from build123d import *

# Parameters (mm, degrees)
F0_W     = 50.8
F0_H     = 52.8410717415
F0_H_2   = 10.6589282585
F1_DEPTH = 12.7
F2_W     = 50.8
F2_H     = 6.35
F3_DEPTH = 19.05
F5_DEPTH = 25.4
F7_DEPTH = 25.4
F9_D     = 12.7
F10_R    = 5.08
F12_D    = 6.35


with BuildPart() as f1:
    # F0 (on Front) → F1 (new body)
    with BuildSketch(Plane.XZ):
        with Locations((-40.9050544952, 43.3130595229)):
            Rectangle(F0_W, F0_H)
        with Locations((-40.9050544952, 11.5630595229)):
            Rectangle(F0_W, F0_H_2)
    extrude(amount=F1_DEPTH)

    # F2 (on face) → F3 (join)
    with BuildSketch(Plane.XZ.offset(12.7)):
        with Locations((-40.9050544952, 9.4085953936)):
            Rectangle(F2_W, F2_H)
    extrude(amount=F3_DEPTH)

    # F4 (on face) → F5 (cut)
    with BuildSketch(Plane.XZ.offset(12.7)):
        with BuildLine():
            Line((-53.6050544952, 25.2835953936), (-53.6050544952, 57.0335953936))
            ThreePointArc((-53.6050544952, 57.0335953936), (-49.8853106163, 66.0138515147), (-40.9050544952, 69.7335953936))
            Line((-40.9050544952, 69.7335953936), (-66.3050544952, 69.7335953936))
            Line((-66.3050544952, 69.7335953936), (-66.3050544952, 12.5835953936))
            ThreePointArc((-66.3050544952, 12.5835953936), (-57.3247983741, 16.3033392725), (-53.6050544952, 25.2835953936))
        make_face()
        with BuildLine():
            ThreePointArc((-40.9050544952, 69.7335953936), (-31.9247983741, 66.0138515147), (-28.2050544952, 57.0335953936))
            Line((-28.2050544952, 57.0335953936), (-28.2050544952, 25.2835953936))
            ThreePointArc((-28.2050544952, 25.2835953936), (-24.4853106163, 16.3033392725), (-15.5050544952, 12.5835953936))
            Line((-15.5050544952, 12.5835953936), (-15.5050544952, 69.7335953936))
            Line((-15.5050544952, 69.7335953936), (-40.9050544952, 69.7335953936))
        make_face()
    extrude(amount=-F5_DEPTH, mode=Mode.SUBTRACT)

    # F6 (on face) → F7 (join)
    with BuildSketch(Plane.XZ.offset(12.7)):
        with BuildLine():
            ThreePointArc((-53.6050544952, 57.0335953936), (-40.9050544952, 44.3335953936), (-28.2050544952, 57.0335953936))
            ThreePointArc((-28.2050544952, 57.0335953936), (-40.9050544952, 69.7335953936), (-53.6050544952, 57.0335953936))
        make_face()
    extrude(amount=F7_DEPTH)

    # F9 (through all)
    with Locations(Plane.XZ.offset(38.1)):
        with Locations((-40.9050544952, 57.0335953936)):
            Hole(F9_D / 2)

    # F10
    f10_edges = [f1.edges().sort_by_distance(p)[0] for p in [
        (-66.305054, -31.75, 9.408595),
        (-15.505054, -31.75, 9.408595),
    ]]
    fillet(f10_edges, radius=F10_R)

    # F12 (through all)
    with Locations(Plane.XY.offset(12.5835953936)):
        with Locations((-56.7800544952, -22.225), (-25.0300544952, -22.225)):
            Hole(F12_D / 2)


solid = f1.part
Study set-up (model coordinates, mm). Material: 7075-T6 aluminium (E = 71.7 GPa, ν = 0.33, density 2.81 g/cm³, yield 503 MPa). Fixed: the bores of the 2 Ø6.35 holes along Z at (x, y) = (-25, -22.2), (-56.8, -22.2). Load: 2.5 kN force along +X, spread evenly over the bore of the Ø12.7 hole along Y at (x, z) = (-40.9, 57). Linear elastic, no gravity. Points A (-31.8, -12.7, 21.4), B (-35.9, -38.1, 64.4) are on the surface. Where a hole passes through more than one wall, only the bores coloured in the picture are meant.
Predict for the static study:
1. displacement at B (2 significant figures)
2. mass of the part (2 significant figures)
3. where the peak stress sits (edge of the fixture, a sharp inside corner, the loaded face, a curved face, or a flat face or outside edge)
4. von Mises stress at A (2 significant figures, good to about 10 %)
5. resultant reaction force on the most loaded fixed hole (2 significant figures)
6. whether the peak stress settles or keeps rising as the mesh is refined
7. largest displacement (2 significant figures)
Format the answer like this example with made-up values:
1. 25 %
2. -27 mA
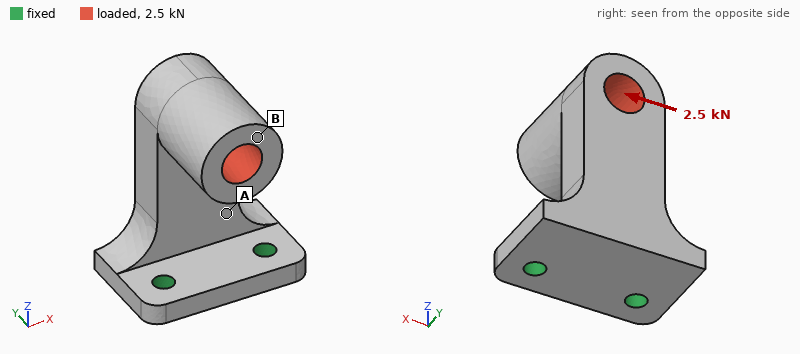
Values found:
1. 0.39 mm
2. 100 g
3. edge of the fixture
4. 91 MPa
5. 3.7 kN
6. keeps rising
7. 0.41 mm
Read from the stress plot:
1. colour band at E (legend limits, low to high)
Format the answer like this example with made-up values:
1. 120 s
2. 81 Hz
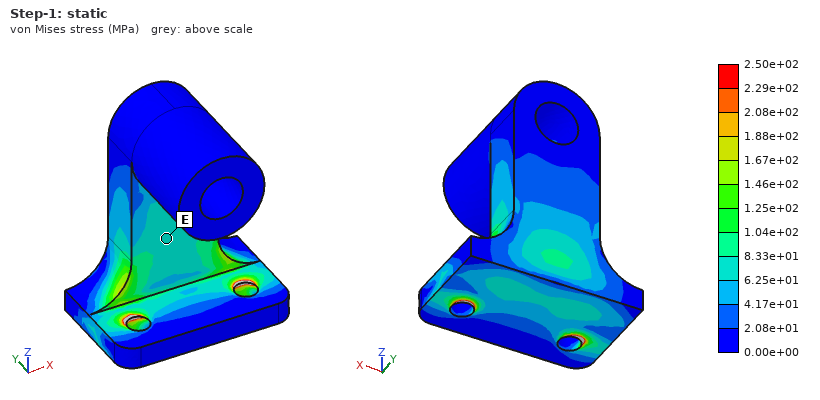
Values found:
1. 6.25e+01 to 8.33e+01 MPa
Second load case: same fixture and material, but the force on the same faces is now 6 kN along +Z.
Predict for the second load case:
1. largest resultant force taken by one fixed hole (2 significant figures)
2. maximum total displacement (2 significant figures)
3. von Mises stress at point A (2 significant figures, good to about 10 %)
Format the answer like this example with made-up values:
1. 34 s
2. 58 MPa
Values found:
1. 3.0 kN
2. 0.70 mm
3. 120 MPa
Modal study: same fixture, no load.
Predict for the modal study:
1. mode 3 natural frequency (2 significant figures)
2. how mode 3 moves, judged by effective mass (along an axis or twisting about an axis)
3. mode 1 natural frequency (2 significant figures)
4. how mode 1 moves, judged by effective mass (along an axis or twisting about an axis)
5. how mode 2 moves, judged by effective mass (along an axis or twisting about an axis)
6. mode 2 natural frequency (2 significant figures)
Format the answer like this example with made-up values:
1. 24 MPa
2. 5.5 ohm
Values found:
1. 4400 Hz
2. along Z
3. 1000 Hz
4. along Y
5. along X
6. 2200 Hz
